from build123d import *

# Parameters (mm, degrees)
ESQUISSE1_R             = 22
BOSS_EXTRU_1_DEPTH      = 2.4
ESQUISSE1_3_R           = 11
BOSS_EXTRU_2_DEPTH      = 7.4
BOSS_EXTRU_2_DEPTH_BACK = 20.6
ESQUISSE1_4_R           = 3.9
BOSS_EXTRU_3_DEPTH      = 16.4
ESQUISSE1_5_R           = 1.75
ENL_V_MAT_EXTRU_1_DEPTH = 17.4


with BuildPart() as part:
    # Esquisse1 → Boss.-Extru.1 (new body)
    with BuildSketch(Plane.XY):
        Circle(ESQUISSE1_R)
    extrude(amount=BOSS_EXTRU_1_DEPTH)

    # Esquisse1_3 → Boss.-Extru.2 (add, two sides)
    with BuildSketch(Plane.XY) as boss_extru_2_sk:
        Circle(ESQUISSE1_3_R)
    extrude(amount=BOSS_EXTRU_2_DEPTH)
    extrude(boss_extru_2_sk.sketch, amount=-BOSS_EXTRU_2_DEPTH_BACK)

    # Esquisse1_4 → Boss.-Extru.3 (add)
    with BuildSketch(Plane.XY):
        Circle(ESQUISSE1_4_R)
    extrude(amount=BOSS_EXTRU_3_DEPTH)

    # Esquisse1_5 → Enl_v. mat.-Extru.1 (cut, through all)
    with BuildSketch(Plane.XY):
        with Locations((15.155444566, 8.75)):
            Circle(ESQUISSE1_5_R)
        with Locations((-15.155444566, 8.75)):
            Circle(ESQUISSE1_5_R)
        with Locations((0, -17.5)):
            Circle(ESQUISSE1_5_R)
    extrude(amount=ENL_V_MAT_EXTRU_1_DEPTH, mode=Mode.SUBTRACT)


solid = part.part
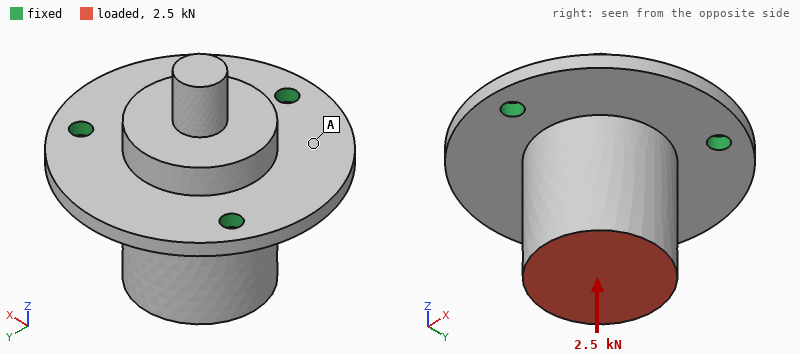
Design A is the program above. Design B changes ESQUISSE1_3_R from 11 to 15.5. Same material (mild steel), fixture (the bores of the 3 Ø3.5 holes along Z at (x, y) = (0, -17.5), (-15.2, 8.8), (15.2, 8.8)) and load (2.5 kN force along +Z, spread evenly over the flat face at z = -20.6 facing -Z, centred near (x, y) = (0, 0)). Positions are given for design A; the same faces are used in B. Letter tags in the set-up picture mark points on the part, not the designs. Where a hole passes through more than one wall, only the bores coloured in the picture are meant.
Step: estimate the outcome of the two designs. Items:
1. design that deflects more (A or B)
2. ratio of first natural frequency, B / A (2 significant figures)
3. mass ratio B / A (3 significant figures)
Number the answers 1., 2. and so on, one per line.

1. A
2. 1.7
3. 1.70
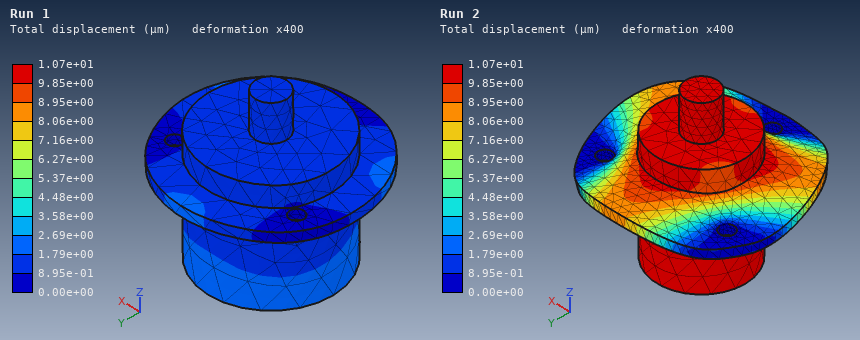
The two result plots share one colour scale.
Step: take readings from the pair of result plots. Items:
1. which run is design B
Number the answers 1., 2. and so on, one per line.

1. Run 1
